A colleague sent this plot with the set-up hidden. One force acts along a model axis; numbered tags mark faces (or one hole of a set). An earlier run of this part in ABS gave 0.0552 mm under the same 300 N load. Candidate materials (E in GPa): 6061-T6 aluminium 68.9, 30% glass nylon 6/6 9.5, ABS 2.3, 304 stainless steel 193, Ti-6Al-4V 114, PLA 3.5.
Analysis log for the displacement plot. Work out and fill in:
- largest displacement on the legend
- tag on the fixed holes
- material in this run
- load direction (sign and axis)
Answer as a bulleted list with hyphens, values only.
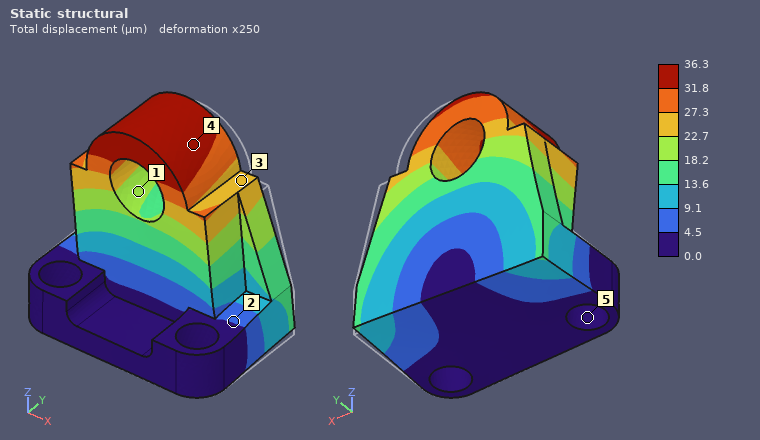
- 36.3 µm
- 5
- PLA
- -X
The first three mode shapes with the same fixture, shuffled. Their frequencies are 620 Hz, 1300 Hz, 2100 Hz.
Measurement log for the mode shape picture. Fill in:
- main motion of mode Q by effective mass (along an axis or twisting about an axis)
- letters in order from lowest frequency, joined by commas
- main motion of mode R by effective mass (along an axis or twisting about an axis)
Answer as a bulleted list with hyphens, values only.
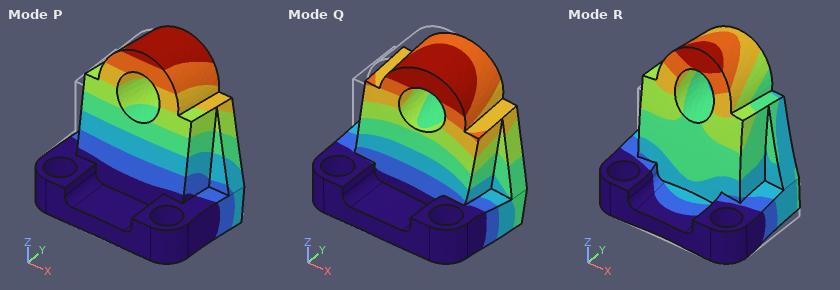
- along X
- P, Q, R
- along Z
